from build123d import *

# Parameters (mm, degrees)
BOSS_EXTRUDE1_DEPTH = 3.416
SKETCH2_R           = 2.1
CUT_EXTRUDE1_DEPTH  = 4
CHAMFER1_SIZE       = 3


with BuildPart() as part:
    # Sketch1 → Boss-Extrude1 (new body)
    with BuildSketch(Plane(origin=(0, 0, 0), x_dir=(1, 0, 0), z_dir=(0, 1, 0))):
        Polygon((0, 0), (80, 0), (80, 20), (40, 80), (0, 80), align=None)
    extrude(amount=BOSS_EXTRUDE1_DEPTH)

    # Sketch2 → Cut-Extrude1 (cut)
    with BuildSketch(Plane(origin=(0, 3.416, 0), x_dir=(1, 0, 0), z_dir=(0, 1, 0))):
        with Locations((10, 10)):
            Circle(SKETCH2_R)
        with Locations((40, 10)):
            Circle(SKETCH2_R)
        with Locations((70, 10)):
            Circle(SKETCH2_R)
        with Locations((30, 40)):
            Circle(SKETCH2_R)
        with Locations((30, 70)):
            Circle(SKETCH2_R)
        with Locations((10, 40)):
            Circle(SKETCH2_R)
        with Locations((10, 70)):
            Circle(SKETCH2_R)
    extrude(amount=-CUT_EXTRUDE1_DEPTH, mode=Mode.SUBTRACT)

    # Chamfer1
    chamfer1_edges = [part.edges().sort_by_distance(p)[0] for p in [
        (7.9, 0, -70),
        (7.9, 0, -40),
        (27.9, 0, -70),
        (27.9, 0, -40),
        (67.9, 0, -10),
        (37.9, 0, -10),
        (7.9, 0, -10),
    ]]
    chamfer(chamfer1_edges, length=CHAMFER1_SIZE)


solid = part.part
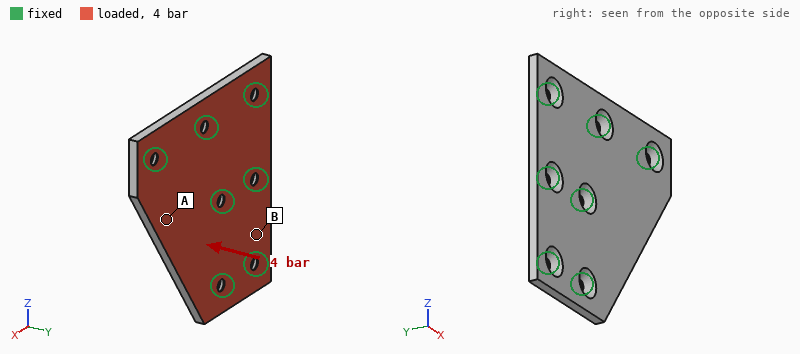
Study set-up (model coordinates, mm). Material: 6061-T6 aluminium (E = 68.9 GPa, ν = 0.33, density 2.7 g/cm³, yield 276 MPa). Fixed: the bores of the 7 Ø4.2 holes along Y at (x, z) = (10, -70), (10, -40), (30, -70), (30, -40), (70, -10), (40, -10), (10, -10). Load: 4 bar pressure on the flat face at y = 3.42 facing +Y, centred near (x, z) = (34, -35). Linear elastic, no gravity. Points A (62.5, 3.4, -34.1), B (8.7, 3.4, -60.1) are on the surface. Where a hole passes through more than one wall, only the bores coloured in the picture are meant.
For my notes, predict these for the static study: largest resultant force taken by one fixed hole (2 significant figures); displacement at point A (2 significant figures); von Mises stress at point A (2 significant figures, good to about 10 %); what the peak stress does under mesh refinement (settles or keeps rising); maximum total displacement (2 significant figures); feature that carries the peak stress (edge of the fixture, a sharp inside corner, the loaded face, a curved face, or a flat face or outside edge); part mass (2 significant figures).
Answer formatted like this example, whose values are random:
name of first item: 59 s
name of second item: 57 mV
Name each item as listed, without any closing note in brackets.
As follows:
largest resultant force taken by one fixed hole: 670 N
displacement at point A: 0.11 mm
von Mises stress at point A: 24 MPa
what the peak stress does under mesh refinement: keeps rising
maximum total displacement: 0.15 mm
feature that carries the peak stress: edge of the fixture
part mass: 45 g
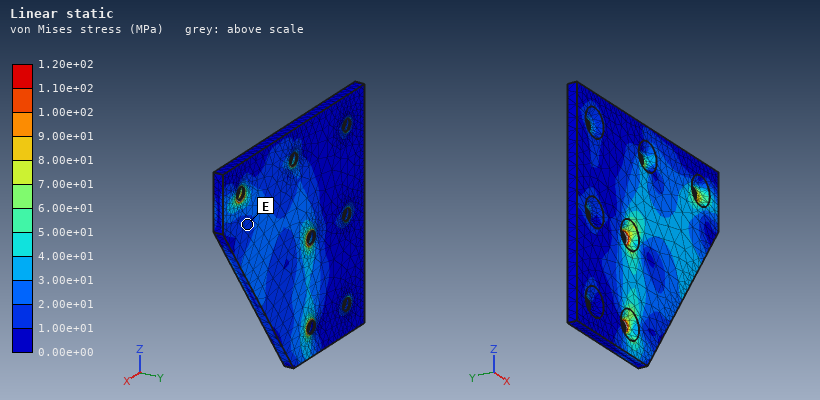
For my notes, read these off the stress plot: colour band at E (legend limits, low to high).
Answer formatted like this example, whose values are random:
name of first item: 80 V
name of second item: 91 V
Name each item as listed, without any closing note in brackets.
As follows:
colour band at E: 1.00e+01 to 2.00e+01 MPa
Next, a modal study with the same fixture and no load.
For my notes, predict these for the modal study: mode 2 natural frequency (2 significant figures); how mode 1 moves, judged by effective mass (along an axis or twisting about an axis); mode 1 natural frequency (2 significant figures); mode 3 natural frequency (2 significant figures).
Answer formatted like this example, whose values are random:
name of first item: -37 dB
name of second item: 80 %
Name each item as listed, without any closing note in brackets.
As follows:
mode 2 natural frequency: 7200 Hz
how mode 1 moves, judged by effective mass: along Y
mode 1 natural frequency: 3500 Hz
mode 3 natural frequency: 11 kHz
